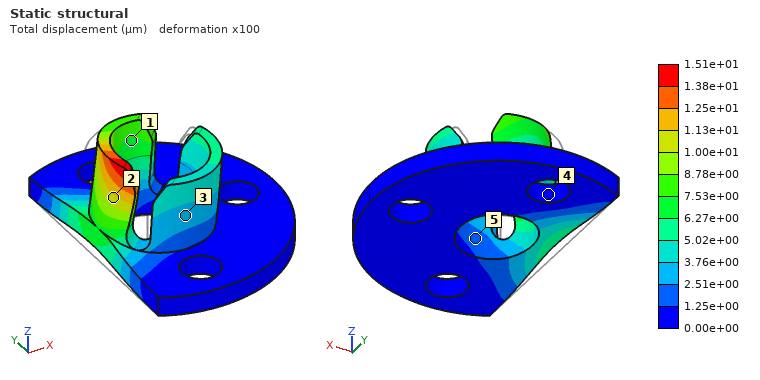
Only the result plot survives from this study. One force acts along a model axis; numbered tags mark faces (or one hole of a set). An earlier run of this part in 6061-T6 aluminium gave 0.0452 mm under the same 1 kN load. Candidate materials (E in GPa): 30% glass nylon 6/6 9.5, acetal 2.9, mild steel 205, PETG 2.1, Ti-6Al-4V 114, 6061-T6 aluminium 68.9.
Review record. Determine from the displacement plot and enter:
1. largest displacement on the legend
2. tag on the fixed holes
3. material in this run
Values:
1.51e+01 µm
4
mild steel
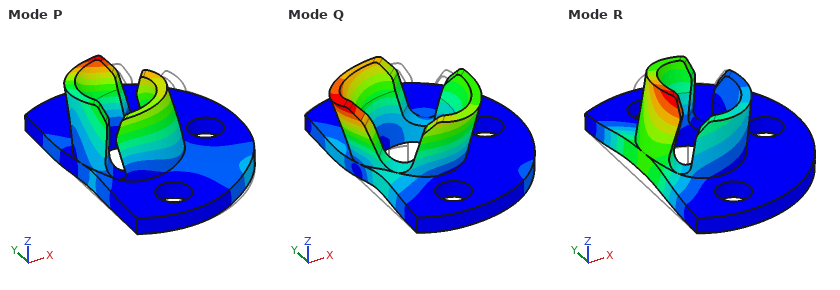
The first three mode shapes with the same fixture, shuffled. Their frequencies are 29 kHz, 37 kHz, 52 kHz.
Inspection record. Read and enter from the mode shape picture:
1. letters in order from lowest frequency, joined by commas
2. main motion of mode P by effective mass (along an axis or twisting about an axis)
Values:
R, Q, P
along Y
